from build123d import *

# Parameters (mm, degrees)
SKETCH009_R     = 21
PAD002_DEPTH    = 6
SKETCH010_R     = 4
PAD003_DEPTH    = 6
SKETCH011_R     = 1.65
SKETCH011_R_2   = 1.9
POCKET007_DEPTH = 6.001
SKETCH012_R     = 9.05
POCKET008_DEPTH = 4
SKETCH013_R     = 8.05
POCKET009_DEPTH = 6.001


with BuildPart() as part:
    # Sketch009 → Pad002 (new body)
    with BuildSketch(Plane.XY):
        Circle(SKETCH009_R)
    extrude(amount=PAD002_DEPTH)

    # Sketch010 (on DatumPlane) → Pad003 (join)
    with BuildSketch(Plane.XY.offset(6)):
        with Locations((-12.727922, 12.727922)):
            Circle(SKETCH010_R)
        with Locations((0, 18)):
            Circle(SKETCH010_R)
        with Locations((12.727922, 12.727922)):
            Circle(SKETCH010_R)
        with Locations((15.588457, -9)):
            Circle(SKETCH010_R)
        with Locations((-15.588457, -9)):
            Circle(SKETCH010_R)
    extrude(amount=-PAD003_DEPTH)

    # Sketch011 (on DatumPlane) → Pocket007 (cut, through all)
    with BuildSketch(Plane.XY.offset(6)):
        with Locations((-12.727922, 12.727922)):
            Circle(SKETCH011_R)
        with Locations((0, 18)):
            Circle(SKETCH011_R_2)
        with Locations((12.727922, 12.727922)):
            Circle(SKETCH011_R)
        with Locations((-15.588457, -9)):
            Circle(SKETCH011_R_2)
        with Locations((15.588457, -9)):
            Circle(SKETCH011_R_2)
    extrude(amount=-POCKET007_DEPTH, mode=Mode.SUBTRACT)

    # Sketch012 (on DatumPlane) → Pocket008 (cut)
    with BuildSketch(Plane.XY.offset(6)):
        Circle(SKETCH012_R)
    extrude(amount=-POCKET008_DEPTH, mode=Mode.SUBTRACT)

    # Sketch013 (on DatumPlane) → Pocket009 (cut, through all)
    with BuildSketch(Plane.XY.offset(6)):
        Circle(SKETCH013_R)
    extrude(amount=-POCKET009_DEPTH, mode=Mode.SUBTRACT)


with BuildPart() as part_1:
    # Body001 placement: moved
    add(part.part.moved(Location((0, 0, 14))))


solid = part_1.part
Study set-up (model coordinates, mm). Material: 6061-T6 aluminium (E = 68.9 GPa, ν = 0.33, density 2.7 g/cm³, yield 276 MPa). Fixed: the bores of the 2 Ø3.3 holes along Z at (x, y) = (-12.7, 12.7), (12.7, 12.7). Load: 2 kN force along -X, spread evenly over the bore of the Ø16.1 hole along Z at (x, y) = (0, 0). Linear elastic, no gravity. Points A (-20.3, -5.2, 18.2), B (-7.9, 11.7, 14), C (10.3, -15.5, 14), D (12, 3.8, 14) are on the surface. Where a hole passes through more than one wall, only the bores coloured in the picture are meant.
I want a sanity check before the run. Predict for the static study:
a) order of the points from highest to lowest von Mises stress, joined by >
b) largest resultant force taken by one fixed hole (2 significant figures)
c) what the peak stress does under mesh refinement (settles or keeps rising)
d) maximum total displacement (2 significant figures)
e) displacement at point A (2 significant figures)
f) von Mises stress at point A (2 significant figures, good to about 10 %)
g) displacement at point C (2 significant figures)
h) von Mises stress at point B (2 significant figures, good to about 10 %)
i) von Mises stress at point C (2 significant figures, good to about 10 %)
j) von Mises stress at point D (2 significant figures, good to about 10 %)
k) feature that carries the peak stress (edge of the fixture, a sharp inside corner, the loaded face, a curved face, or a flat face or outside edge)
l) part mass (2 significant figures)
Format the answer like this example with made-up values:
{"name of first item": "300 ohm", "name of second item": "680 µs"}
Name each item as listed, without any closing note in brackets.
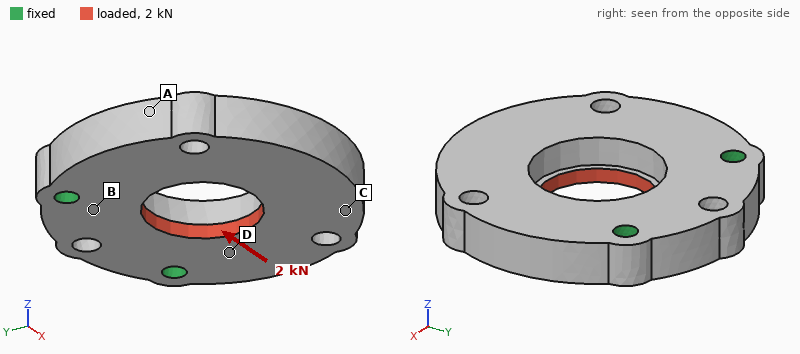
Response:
{"order of the points from highest to lowest von Mises stress, joined by >": "D > B > A > C", "largest resultant force taken by one fixed hole": "1.3 kN", "what the peak stress does under mesh refinement": "keeps rising", "maximum total displacement": "27 µm", "displacement at point A": "21 µm", "von Mises stress at point A": "13 MPa", "displacement at point C": "26 µm", "von Mises stress at point B": "23 MPa", "von Mises stress at point C": "7.0 MPa", "von Mises stress at point D": "35 MPa", "feature that carries the peak stress": "edge of the fixture", "part mass": "18 g"}
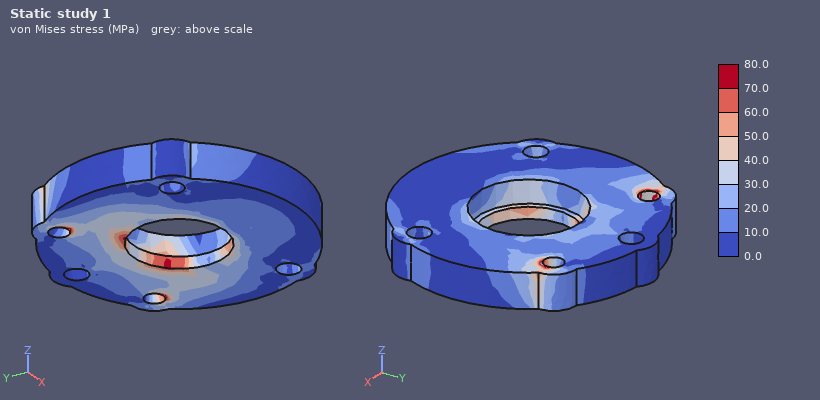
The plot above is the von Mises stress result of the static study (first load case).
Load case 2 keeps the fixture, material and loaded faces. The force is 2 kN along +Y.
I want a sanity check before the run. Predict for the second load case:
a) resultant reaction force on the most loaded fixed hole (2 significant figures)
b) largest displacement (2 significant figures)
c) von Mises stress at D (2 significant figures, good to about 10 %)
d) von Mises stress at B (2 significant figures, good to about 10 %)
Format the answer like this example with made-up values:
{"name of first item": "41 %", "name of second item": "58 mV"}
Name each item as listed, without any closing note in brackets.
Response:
{"resultant reaction force on the most loaded fixed hole": "1.0 kN", "largest displacement": "45 µm", "von Mises stress at D": "29 MPa", "von Mises stress at B": "19 MPa"}
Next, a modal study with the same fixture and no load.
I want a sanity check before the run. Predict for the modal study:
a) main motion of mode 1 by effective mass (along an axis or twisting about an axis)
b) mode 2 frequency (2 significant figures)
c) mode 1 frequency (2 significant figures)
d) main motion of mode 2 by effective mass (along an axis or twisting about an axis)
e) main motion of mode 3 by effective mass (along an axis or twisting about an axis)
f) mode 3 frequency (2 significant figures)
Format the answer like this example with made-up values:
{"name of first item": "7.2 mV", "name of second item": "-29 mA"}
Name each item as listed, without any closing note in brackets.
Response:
{"main motion of mode 1 by effective mass": "along Z", "mode 2 frequency": "9900 Hz", "mode 1 frequency": "4100 Hz", "main motion of mode 2 by effective mass": "twisting about Y", "main motion of mode 3 by effective mass": "along X", "mode 3 frequency": "12 kHz"}
